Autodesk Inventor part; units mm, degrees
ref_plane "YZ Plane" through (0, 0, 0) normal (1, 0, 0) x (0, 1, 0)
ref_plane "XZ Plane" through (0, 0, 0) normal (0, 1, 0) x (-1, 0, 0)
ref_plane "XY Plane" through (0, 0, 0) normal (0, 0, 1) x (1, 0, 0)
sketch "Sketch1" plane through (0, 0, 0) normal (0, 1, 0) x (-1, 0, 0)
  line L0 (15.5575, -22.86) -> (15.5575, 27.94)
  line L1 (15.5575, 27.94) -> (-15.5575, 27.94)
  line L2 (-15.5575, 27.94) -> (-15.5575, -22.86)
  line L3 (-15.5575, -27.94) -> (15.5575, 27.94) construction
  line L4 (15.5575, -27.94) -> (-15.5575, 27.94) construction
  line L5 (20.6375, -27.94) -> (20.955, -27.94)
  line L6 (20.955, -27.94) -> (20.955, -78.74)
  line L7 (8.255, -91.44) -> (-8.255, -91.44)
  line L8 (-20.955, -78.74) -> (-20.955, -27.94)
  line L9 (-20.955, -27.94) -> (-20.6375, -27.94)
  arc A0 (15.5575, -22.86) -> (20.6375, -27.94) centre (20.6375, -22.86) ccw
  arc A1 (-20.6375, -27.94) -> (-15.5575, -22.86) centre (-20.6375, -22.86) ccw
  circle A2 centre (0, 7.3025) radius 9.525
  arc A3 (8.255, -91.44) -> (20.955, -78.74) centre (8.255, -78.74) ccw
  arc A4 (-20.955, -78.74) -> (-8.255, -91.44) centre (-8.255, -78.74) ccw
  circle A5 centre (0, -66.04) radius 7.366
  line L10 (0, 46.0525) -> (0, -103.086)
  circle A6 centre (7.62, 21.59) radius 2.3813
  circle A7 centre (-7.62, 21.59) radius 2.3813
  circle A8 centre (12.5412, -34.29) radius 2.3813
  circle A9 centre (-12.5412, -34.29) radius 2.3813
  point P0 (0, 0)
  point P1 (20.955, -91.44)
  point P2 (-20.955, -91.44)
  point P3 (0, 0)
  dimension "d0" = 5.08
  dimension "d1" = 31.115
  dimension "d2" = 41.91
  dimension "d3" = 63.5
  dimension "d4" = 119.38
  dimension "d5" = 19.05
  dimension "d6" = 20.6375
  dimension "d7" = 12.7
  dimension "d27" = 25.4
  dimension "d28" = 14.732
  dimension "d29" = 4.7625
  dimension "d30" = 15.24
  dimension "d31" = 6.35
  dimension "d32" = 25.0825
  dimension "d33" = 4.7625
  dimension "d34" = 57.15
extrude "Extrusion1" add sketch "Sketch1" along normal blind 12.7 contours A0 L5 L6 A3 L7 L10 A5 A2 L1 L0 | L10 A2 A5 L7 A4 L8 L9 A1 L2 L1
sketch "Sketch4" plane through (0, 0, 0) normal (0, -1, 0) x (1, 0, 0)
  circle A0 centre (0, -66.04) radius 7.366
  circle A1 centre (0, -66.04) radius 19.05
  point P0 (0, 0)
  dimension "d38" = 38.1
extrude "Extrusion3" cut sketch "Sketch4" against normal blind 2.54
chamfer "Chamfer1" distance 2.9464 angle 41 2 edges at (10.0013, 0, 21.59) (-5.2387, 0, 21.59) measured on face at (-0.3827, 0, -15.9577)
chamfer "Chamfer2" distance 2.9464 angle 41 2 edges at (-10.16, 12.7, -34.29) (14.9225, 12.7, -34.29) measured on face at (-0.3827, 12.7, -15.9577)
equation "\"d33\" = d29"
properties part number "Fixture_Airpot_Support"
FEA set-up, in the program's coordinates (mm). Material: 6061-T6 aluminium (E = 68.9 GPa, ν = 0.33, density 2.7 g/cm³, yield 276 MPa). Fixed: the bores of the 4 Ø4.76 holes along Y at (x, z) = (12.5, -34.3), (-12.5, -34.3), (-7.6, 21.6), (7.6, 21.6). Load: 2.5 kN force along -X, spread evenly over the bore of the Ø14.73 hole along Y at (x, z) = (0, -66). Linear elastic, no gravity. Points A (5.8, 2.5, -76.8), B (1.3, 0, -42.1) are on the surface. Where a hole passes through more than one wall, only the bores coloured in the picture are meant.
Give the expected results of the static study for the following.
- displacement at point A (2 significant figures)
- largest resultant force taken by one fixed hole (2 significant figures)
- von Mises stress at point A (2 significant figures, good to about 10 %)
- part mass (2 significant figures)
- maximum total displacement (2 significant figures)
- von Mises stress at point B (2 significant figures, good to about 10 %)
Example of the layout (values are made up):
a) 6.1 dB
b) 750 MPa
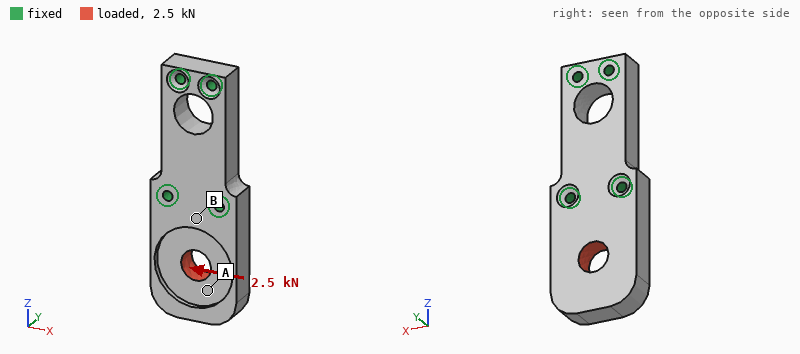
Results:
a) 23 µm
b) 3.0 kN
c) 5.3 MPa
d) 120 g
e) 28 µm
f) 15 MPa
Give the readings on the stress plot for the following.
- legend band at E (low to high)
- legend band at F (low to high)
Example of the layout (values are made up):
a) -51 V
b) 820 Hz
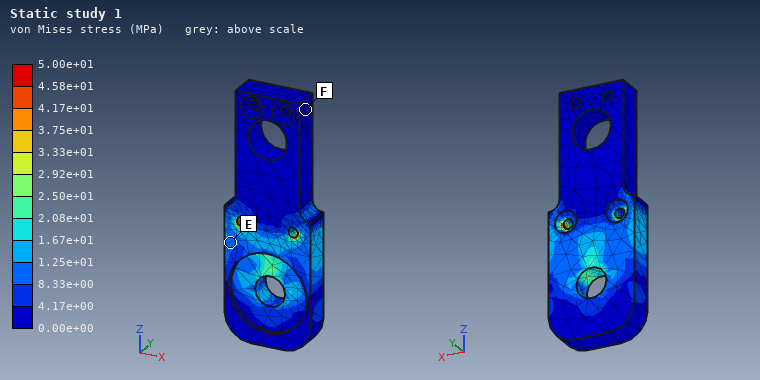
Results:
a) 8.33e+00 to 1.25e+01 MPa
b) 0.00e+00 to 4.17e+00 MPa
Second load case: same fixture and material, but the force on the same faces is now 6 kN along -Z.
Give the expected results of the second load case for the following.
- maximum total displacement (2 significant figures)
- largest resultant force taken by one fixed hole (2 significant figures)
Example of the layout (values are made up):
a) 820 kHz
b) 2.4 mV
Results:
a) 25 µm
b) 2.9 kN
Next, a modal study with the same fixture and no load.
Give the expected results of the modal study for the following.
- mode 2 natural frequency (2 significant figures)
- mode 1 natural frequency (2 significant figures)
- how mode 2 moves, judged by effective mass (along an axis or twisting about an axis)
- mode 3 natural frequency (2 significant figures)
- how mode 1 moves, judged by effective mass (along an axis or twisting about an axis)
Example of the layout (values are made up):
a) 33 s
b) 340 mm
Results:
a) 6800 Hz
b) 2800 Hz
c) along X
d) 7700 Hz
e) along Y
